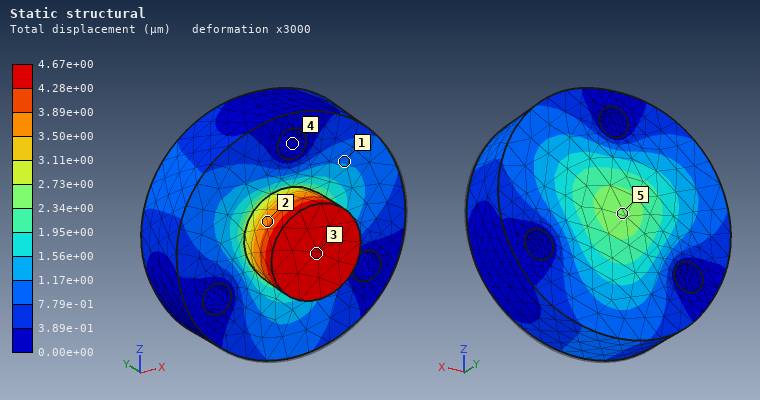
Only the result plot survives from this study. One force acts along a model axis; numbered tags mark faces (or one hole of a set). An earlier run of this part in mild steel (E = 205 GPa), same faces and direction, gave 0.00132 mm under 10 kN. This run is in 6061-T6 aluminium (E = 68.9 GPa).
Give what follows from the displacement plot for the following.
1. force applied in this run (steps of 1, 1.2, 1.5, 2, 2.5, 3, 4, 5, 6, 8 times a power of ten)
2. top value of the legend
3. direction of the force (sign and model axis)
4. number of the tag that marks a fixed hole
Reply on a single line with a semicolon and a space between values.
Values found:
12 kN; 4.67e+00 µm; +Y; 4
